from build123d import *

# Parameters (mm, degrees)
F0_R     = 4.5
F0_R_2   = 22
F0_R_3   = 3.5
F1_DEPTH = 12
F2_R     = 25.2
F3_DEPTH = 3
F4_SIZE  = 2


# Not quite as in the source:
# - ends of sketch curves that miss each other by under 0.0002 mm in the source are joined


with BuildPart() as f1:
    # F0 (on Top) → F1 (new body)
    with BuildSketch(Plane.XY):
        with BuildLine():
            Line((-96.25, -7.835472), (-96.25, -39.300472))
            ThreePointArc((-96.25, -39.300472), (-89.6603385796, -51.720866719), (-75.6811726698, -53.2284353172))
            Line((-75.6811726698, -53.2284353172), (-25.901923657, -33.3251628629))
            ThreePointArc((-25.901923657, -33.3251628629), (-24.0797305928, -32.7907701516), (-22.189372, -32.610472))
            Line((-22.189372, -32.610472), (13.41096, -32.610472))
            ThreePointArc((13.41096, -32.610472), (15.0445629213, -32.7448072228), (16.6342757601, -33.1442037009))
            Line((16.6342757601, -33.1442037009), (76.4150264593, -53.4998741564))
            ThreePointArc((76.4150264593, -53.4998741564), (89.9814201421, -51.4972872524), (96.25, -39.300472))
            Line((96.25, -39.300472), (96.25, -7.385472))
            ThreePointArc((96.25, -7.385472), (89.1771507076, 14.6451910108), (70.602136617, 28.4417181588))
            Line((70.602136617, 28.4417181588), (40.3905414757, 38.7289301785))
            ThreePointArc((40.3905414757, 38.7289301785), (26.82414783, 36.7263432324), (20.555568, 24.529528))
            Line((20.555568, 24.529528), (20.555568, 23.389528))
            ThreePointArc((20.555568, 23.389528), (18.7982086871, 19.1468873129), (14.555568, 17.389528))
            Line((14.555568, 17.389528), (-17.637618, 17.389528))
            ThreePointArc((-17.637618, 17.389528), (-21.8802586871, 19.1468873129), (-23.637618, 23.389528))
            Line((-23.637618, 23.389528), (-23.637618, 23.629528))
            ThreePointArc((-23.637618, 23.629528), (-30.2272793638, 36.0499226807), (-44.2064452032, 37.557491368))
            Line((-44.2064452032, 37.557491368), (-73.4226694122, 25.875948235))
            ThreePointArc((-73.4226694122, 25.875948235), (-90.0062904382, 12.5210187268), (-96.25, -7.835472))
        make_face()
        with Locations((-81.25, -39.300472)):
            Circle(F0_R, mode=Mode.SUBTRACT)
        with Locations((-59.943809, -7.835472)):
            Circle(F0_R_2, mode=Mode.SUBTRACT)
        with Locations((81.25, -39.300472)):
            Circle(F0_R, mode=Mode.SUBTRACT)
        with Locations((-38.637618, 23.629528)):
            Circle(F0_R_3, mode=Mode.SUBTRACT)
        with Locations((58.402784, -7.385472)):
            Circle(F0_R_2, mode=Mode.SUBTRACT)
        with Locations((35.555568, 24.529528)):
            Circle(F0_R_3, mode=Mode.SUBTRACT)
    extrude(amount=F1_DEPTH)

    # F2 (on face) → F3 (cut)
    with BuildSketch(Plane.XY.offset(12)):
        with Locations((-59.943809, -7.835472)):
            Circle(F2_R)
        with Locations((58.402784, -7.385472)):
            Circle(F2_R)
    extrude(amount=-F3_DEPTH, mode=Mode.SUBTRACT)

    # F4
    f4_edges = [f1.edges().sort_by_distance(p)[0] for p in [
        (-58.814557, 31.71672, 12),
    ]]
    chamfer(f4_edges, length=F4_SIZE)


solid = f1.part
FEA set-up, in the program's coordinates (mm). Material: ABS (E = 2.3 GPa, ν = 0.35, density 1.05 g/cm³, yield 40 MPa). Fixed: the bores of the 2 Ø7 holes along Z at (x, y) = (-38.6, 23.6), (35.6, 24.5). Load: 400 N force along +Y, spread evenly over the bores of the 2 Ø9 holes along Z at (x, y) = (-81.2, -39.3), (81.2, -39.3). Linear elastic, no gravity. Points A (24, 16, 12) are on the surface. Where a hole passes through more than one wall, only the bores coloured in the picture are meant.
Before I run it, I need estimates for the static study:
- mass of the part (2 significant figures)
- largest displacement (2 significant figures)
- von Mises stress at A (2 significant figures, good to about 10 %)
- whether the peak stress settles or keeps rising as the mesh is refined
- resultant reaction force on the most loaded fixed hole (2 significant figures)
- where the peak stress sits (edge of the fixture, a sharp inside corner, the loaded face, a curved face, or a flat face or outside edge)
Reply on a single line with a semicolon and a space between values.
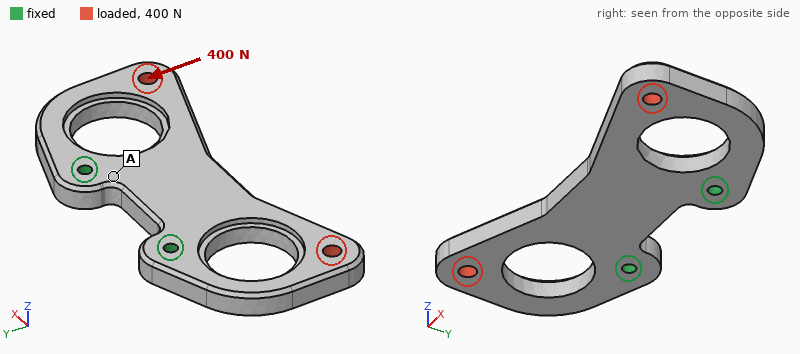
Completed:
120 g; 0.18 mm; 0.68 MPa; keeps rising; 260 N; edge of the fixture
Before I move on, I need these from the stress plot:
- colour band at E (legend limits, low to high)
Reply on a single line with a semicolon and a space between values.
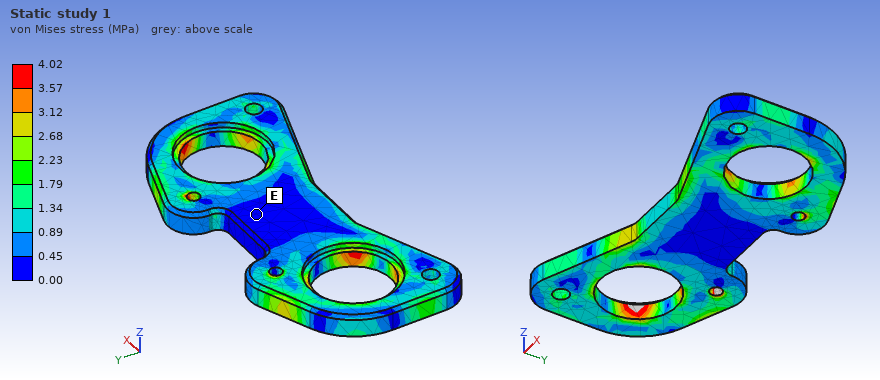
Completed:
0.00 to 0.45 MPa
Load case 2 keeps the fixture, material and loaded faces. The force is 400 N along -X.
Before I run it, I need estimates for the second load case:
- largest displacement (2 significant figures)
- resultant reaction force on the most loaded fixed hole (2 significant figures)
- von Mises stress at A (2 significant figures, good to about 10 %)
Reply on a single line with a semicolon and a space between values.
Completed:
0.15 mm; 370 N; 1.2 MPa
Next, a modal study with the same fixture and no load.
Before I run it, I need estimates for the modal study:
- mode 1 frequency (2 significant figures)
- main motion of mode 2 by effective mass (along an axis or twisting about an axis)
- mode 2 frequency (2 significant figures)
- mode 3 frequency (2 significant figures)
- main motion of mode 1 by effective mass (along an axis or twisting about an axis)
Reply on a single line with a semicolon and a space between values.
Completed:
320 Hz; twisting about Y; 360 Hz; 680 Hz; along Z
